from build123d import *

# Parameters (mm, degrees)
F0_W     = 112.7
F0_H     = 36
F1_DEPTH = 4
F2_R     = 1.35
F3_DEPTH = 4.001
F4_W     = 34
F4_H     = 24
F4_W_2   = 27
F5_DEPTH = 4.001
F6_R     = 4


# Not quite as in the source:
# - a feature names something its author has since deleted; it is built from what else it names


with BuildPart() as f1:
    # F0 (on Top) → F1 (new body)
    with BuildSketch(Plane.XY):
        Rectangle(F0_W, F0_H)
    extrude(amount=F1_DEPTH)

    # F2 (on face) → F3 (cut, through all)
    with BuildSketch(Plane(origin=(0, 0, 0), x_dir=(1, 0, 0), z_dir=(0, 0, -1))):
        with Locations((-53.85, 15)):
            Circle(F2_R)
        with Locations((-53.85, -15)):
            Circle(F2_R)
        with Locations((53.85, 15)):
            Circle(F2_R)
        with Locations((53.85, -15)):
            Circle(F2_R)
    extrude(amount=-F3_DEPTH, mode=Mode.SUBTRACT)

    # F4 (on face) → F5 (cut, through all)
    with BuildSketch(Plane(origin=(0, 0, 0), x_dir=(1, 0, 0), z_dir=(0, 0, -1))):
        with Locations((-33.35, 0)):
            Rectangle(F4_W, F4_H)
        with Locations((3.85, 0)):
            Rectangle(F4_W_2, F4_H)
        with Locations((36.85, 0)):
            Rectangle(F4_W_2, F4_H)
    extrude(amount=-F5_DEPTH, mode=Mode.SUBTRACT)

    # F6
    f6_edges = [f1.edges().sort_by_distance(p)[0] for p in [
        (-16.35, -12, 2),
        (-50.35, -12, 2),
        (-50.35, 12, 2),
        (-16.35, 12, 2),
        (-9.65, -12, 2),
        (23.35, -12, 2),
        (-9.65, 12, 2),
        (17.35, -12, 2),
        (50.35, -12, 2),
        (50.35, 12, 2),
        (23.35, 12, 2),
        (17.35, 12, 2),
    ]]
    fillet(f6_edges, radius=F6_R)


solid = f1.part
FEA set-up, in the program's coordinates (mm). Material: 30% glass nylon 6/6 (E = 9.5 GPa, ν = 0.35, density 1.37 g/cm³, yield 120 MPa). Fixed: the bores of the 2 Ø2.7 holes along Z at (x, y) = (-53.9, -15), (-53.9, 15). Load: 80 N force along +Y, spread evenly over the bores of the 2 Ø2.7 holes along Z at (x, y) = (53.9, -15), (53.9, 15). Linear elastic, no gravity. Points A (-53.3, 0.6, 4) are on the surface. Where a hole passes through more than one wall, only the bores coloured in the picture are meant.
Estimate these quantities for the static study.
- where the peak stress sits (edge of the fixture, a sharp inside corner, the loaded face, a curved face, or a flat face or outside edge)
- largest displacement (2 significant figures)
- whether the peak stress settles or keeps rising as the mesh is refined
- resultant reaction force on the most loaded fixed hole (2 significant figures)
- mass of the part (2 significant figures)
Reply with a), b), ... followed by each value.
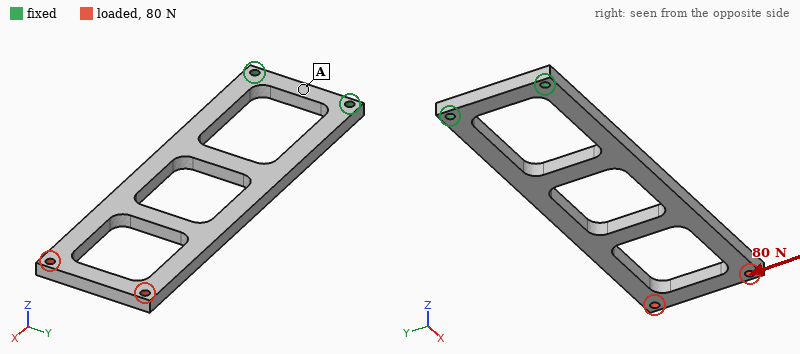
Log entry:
a) edge of the fixture
b) 1.1 mm
c) keeps rising
d) 250 N
e) 11 g
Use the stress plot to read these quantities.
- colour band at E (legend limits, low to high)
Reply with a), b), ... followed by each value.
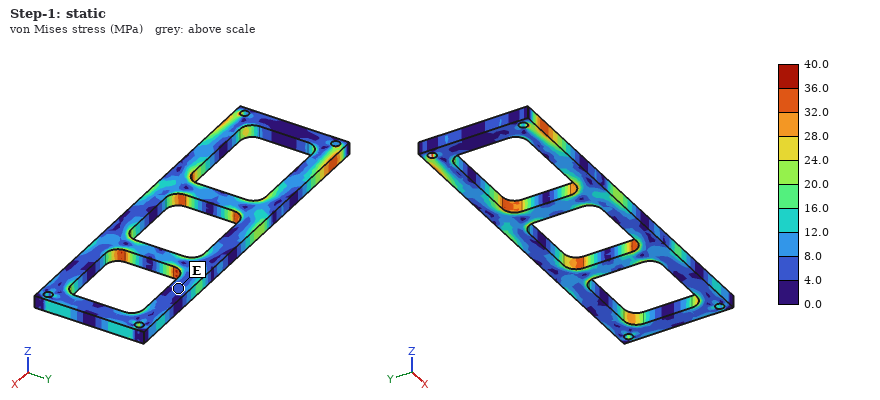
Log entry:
a) 4.0 to 8.0 MPa
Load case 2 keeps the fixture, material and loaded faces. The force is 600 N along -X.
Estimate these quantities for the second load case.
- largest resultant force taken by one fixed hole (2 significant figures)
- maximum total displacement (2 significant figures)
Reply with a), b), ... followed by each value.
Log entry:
a) 300 N
b) 0.15 mm
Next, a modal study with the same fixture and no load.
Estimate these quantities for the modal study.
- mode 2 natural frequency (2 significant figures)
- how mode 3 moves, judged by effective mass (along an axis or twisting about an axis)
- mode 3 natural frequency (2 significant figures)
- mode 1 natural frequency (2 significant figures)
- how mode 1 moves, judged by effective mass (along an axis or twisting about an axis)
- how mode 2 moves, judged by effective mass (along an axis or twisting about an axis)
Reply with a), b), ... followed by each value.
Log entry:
a) 560 Hz
b) along Y
c) 670 Hz
d) 120 Hz
e) along Z
f) twisting about X
